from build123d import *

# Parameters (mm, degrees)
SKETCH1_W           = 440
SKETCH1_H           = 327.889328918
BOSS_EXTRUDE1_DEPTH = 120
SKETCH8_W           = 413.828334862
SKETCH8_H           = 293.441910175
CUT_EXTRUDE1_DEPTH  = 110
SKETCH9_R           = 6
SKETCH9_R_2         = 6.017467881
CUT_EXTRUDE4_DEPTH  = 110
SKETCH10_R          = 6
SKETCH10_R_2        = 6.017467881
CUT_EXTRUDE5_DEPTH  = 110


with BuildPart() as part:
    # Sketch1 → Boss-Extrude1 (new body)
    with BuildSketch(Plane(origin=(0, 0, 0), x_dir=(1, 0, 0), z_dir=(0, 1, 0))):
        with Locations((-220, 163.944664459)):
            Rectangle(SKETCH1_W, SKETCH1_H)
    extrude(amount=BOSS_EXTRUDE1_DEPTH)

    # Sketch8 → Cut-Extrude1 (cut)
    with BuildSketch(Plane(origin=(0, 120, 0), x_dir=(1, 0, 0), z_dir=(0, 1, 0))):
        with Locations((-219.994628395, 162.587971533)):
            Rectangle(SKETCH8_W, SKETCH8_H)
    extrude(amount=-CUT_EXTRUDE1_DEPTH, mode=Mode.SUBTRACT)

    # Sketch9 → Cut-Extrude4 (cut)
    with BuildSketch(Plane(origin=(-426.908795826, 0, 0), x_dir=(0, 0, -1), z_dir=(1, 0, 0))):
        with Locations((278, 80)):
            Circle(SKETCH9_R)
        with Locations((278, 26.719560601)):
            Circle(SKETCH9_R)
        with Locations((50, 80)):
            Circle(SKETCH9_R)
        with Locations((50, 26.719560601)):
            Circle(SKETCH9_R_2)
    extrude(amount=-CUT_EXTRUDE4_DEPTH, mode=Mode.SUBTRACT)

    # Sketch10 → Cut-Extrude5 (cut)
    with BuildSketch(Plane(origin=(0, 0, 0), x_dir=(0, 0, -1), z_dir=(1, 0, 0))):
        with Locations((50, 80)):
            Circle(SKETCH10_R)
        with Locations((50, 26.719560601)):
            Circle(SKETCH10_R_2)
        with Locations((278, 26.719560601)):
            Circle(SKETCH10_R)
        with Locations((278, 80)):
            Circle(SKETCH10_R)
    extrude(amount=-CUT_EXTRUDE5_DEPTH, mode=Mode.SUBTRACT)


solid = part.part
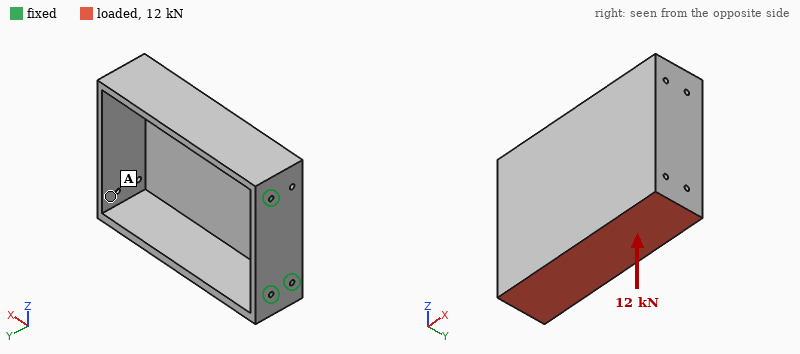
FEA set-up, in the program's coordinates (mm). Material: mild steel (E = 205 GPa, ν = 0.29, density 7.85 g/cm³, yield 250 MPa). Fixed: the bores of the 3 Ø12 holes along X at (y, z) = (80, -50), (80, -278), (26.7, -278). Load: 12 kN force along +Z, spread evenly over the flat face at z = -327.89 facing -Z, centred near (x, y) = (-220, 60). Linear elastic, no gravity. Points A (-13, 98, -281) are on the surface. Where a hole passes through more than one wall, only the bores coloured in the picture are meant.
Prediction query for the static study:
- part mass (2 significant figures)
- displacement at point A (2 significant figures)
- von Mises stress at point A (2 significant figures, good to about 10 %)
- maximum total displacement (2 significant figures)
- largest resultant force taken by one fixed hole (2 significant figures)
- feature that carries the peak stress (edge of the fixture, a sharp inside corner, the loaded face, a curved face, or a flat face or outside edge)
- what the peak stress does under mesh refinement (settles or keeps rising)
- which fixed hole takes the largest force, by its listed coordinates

31 kg
0.71 mm
16 MPa
1.3 mm
9.9 kN
edge of the fixture
keeps rising
(80, -50)
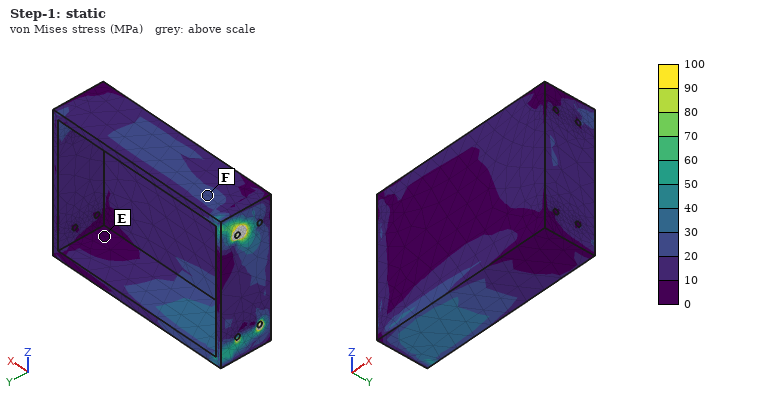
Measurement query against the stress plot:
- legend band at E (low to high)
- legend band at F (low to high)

0 to 10 MPa
20 to 30 MPa
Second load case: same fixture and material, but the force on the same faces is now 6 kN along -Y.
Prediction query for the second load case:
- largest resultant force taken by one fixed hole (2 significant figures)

17 kN
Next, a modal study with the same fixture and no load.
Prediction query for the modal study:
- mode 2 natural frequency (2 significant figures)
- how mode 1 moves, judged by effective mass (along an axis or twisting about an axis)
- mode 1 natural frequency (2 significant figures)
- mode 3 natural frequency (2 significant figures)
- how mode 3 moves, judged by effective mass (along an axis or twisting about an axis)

170 Hz
along Y
91 Hz
410 Hz
along Z
